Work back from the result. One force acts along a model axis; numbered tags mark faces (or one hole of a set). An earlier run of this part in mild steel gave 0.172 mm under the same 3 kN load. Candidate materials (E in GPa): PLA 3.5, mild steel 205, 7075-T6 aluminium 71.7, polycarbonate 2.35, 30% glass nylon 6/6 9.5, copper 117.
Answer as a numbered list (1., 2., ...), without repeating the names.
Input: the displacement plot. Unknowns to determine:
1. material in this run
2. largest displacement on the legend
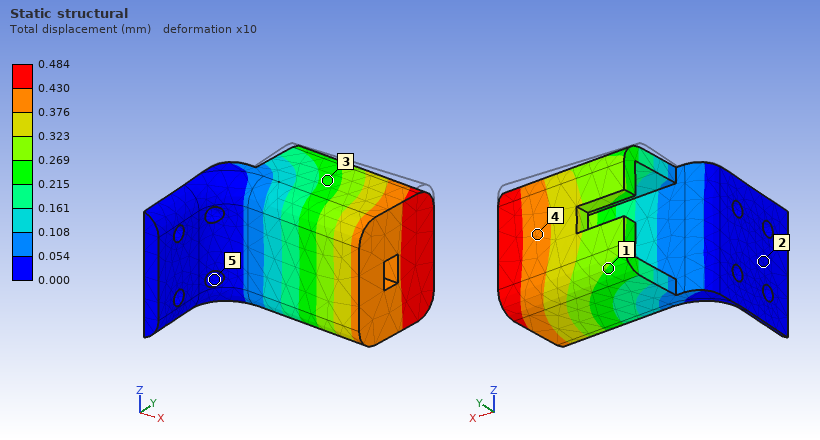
1. 7075-T6 aluminium
2. 0.484 mm
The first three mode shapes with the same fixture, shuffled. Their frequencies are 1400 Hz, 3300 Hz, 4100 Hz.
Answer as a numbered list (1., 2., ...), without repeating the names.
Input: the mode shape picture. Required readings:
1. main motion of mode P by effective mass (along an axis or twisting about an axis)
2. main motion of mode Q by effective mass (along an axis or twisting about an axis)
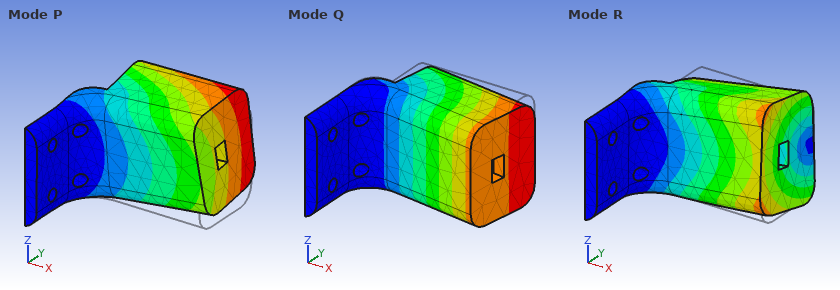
1. along Z
2. along Y
